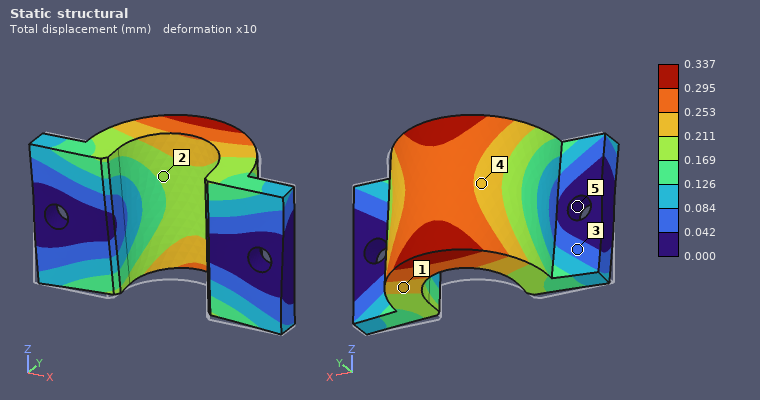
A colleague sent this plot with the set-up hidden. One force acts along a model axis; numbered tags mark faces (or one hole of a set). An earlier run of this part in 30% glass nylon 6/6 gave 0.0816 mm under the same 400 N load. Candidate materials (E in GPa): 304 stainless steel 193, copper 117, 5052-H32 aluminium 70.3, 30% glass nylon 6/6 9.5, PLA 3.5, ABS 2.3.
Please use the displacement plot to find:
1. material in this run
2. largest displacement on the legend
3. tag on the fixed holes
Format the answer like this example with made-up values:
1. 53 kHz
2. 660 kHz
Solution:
1. ABS
2. 0.337 mm
3. 5
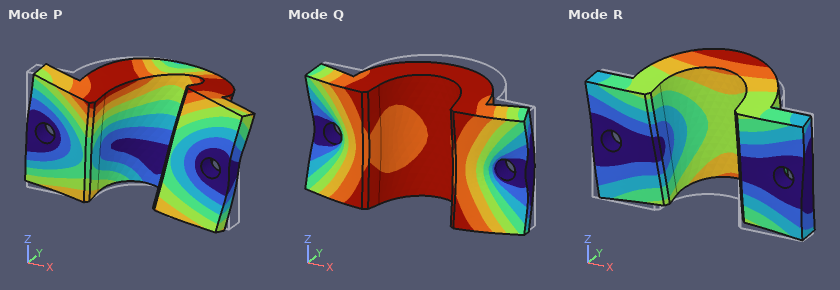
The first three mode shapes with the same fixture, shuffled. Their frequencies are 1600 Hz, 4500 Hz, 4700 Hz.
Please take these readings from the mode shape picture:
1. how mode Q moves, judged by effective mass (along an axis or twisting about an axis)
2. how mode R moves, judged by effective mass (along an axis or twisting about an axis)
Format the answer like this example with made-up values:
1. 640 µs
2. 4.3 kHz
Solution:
1. along Y
2. along Z
